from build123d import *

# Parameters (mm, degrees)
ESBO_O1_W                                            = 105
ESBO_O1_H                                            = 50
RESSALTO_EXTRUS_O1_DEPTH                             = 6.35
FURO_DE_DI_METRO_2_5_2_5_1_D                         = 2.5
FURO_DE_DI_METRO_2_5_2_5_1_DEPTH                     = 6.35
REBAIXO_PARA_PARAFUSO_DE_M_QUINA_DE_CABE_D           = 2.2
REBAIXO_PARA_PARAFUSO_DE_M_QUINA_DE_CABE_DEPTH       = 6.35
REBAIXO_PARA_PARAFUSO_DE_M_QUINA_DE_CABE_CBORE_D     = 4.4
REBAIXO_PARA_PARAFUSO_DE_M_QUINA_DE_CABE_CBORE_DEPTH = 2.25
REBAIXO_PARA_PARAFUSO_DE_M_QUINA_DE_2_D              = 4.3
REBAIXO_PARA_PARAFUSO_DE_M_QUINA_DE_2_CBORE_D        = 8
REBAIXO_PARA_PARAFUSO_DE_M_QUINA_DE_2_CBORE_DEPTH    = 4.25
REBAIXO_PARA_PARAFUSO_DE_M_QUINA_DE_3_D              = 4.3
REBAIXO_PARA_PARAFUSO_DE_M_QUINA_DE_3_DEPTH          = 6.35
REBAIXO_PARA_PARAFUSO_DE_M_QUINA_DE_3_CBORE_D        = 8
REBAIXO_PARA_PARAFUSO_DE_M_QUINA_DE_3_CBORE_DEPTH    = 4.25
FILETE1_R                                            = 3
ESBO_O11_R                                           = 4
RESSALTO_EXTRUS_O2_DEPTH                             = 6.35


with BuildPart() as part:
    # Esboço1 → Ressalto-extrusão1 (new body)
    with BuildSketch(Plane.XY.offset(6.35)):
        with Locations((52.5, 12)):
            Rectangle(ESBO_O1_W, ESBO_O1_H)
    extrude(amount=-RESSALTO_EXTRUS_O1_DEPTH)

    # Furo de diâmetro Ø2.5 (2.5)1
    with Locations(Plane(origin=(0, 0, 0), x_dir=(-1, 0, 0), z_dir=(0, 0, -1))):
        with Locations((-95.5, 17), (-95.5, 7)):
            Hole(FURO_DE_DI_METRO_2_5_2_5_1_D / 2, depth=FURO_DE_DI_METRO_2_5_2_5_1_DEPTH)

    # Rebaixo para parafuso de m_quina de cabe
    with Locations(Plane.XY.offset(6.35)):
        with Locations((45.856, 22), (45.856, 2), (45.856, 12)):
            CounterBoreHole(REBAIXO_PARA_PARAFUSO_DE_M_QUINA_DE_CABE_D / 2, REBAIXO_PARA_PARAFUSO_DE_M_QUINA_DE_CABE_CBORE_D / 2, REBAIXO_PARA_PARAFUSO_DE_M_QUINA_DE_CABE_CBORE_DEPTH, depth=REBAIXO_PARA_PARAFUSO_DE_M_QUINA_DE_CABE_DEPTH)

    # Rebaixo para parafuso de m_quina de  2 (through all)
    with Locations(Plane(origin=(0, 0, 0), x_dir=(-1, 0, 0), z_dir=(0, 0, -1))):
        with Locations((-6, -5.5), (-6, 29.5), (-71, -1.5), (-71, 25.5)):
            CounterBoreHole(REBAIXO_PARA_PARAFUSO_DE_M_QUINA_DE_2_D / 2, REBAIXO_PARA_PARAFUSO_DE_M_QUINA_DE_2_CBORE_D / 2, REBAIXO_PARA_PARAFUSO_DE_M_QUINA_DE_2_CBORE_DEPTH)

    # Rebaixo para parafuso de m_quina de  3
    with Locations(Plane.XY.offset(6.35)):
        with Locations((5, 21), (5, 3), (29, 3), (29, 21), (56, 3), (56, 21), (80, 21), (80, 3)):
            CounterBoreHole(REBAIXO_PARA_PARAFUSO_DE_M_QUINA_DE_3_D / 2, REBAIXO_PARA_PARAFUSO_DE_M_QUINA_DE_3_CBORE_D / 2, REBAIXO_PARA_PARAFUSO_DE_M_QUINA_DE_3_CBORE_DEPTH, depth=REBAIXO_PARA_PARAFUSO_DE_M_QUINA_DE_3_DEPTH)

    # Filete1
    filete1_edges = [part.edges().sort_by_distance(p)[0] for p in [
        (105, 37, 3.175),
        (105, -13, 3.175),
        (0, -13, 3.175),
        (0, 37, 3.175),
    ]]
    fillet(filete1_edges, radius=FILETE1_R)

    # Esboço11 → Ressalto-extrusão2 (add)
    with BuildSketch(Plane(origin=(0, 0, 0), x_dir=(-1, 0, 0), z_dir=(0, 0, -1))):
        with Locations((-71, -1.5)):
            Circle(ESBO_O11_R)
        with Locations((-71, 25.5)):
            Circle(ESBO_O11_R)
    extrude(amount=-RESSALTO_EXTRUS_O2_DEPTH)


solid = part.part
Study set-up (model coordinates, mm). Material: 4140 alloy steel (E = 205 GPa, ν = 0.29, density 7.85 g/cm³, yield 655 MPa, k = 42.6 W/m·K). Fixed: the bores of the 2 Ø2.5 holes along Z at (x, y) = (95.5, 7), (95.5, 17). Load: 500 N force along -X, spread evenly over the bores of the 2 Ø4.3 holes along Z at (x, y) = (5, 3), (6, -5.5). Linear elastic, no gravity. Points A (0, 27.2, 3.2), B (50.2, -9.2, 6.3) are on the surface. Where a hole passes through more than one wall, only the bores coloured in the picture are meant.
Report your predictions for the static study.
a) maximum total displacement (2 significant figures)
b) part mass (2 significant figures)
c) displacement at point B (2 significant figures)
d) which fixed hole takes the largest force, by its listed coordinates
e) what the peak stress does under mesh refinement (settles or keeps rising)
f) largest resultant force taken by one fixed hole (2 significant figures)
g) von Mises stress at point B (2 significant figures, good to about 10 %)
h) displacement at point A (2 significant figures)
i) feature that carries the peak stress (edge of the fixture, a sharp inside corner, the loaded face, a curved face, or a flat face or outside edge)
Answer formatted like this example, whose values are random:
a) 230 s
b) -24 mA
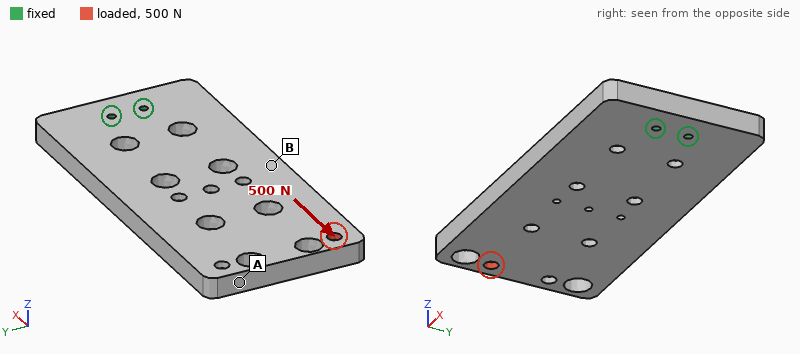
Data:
a) 8.9 µm
b) 240 g
c) 4.1 µm
d) (95.5, 7)
e) keeps rising
f) 810 N
g) 4.4 MPa
h) 8.1 µm
i) edge of the fixture
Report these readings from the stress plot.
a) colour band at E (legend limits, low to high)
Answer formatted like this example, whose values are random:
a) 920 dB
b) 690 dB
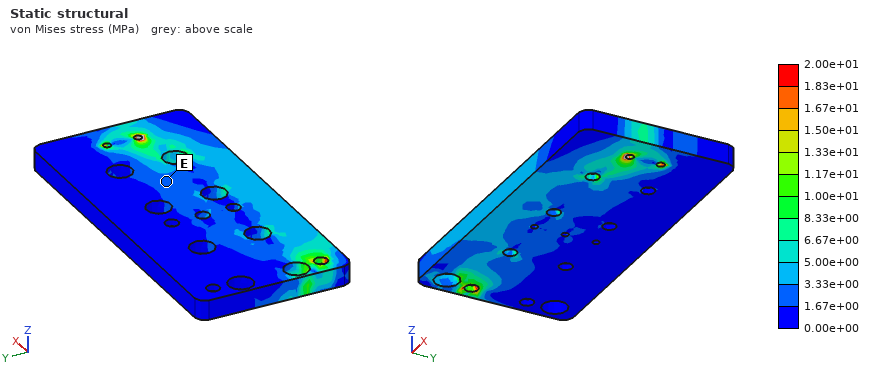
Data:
a) 1.67e+00 to 3.33e+00 MPa
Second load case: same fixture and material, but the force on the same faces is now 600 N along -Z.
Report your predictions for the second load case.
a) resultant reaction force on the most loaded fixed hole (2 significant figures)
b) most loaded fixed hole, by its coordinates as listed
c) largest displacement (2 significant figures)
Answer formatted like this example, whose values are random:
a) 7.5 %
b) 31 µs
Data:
a) 710 N
b) (95.5, 7)
c) 1.00 mm
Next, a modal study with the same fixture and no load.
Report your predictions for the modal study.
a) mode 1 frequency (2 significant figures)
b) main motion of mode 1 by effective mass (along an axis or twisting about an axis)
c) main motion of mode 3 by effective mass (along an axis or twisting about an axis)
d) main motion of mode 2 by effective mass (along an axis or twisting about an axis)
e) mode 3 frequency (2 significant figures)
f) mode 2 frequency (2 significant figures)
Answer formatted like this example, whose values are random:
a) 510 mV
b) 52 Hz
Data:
a) 540 Hz
b) along Z
c) twisting about X
d) along Y
e) 2000 Hz
f) 1800 Hz
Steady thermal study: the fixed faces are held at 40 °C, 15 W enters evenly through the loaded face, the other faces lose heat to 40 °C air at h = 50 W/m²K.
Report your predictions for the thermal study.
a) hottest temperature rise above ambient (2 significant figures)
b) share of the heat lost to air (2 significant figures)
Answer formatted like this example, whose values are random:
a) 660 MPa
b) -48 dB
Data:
a) 78 K
b) 82 %
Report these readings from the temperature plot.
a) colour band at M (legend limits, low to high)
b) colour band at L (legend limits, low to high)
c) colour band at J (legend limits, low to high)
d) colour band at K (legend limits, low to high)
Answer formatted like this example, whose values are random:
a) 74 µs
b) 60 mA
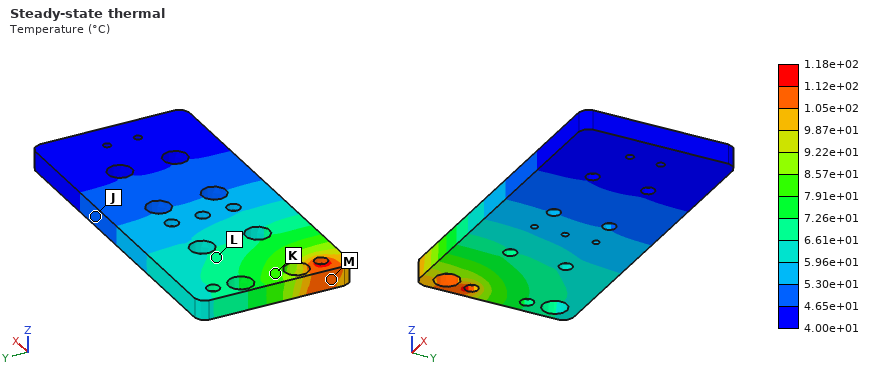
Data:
a) 1.05e+02 to 1.12e+02 °C
b) 6.61e+01 to 7.26e+01 °C
c) 4.65e+01 to 5.30e+01 °C
d) 7.91e+01 to 8.57e+01 °C
